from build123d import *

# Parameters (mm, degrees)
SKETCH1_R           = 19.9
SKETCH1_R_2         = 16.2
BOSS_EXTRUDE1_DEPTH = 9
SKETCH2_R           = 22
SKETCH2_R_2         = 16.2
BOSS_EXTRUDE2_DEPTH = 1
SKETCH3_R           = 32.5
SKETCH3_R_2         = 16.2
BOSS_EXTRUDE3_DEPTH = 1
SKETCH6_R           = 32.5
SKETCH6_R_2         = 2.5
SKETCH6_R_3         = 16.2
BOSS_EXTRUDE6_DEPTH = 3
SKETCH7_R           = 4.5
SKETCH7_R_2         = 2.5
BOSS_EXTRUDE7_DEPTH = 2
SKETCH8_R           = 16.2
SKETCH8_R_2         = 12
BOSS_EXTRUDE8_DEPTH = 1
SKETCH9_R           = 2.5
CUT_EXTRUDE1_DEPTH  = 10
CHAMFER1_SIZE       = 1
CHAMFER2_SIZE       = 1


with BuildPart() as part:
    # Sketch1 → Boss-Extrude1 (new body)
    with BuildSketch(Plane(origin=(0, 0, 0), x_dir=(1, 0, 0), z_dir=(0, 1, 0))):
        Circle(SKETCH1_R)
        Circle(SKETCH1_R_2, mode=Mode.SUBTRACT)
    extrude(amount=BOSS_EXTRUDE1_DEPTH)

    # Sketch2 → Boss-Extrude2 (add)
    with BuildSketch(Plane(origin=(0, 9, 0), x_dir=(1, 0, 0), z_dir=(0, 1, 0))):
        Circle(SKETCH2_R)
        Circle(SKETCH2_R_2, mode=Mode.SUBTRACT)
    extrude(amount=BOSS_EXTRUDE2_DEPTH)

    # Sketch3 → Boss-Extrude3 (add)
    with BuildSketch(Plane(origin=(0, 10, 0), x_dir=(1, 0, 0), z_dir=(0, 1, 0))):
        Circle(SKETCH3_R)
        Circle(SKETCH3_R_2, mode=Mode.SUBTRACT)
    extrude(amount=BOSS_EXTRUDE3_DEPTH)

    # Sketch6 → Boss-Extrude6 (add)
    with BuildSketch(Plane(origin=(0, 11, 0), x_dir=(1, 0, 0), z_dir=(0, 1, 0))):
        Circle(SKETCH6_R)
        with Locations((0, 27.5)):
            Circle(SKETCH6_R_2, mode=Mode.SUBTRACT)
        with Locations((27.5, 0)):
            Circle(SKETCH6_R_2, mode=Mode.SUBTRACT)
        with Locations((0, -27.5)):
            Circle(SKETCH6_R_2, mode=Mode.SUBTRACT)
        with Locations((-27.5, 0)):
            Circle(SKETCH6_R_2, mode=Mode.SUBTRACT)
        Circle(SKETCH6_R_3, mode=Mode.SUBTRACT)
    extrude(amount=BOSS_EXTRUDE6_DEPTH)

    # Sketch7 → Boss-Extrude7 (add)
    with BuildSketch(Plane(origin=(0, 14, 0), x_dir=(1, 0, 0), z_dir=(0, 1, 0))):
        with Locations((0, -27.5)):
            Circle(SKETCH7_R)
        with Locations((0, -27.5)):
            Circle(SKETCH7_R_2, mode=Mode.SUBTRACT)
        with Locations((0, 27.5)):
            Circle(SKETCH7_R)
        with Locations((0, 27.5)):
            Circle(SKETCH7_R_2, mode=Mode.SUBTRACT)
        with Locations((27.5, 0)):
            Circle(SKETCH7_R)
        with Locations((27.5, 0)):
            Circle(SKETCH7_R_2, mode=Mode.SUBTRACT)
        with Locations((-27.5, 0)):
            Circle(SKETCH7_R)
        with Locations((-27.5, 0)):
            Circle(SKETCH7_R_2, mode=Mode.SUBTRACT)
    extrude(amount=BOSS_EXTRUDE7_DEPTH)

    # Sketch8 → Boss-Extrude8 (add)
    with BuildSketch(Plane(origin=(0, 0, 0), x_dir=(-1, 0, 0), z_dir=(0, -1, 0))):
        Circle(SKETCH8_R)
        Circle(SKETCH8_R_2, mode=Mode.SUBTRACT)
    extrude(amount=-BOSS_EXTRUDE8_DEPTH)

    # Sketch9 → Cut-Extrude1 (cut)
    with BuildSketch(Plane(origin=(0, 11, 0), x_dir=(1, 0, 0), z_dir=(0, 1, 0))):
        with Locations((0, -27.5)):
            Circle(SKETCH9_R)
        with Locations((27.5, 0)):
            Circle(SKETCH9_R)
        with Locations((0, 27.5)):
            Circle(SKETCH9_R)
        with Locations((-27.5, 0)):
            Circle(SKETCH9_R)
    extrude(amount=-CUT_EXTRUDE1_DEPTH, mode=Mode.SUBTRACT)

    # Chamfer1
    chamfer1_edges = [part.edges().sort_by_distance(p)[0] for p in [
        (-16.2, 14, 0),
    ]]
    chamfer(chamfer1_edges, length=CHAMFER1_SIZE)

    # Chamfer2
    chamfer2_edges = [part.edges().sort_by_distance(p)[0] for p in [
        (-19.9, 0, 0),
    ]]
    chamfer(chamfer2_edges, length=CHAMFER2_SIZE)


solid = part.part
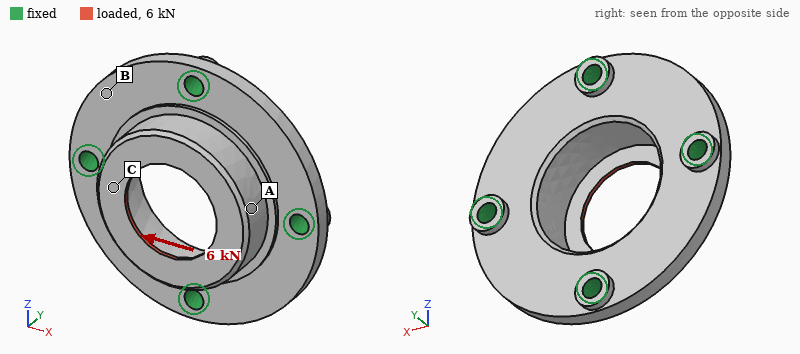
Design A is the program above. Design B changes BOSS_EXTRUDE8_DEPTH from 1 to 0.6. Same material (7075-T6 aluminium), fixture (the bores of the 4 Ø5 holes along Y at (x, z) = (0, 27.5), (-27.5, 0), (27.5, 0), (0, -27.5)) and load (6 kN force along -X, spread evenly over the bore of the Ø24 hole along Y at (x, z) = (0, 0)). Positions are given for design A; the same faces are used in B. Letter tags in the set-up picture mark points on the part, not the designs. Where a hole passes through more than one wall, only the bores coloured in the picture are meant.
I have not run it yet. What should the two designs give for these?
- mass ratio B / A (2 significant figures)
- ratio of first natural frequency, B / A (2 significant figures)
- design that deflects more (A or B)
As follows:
0.99
0.98
B
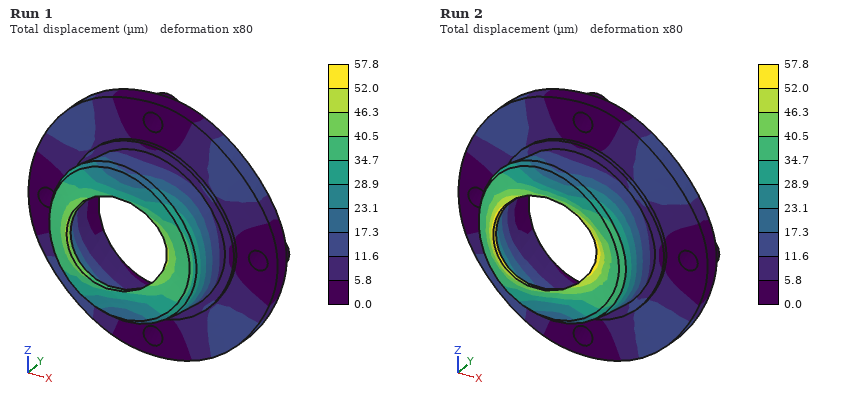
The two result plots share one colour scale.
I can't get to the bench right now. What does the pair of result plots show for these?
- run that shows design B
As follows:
Run 2
